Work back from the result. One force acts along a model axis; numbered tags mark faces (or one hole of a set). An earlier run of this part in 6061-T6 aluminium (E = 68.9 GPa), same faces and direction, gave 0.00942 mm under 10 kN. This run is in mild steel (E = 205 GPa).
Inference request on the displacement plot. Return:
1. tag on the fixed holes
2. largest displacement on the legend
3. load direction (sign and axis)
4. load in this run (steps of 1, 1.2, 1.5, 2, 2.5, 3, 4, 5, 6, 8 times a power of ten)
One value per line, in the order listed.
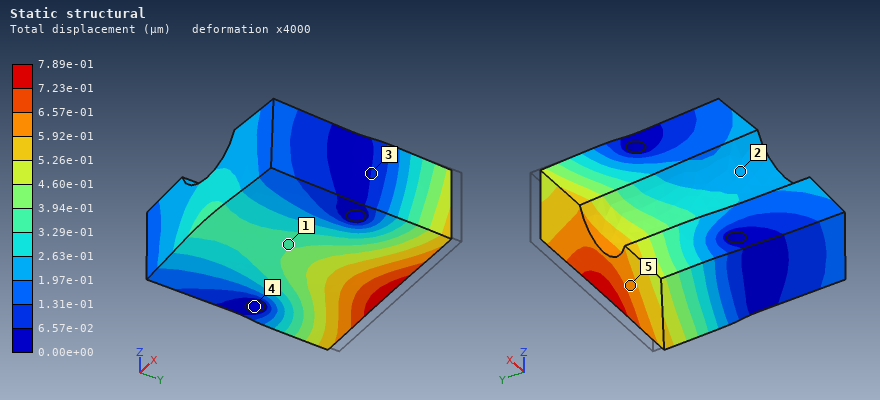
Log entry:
4
7.89e-01 µm
-Y
2.5 kN
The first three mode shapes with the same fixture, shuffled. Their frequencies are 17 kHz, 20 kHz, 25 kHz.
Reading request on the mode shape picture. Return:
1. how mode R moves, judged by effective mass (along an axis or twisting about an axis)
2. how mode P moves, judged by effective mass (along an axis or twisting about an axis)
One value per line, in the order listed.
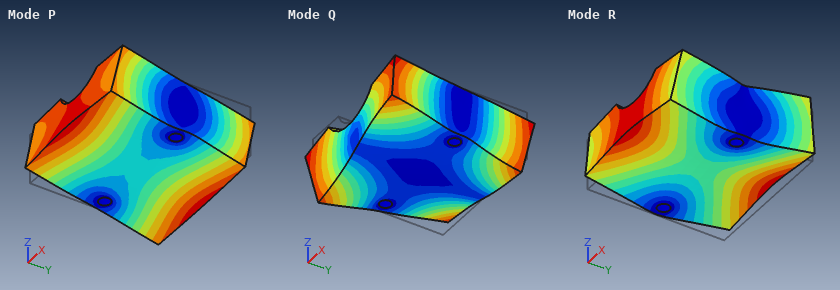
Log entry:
along Z
twisting about X
